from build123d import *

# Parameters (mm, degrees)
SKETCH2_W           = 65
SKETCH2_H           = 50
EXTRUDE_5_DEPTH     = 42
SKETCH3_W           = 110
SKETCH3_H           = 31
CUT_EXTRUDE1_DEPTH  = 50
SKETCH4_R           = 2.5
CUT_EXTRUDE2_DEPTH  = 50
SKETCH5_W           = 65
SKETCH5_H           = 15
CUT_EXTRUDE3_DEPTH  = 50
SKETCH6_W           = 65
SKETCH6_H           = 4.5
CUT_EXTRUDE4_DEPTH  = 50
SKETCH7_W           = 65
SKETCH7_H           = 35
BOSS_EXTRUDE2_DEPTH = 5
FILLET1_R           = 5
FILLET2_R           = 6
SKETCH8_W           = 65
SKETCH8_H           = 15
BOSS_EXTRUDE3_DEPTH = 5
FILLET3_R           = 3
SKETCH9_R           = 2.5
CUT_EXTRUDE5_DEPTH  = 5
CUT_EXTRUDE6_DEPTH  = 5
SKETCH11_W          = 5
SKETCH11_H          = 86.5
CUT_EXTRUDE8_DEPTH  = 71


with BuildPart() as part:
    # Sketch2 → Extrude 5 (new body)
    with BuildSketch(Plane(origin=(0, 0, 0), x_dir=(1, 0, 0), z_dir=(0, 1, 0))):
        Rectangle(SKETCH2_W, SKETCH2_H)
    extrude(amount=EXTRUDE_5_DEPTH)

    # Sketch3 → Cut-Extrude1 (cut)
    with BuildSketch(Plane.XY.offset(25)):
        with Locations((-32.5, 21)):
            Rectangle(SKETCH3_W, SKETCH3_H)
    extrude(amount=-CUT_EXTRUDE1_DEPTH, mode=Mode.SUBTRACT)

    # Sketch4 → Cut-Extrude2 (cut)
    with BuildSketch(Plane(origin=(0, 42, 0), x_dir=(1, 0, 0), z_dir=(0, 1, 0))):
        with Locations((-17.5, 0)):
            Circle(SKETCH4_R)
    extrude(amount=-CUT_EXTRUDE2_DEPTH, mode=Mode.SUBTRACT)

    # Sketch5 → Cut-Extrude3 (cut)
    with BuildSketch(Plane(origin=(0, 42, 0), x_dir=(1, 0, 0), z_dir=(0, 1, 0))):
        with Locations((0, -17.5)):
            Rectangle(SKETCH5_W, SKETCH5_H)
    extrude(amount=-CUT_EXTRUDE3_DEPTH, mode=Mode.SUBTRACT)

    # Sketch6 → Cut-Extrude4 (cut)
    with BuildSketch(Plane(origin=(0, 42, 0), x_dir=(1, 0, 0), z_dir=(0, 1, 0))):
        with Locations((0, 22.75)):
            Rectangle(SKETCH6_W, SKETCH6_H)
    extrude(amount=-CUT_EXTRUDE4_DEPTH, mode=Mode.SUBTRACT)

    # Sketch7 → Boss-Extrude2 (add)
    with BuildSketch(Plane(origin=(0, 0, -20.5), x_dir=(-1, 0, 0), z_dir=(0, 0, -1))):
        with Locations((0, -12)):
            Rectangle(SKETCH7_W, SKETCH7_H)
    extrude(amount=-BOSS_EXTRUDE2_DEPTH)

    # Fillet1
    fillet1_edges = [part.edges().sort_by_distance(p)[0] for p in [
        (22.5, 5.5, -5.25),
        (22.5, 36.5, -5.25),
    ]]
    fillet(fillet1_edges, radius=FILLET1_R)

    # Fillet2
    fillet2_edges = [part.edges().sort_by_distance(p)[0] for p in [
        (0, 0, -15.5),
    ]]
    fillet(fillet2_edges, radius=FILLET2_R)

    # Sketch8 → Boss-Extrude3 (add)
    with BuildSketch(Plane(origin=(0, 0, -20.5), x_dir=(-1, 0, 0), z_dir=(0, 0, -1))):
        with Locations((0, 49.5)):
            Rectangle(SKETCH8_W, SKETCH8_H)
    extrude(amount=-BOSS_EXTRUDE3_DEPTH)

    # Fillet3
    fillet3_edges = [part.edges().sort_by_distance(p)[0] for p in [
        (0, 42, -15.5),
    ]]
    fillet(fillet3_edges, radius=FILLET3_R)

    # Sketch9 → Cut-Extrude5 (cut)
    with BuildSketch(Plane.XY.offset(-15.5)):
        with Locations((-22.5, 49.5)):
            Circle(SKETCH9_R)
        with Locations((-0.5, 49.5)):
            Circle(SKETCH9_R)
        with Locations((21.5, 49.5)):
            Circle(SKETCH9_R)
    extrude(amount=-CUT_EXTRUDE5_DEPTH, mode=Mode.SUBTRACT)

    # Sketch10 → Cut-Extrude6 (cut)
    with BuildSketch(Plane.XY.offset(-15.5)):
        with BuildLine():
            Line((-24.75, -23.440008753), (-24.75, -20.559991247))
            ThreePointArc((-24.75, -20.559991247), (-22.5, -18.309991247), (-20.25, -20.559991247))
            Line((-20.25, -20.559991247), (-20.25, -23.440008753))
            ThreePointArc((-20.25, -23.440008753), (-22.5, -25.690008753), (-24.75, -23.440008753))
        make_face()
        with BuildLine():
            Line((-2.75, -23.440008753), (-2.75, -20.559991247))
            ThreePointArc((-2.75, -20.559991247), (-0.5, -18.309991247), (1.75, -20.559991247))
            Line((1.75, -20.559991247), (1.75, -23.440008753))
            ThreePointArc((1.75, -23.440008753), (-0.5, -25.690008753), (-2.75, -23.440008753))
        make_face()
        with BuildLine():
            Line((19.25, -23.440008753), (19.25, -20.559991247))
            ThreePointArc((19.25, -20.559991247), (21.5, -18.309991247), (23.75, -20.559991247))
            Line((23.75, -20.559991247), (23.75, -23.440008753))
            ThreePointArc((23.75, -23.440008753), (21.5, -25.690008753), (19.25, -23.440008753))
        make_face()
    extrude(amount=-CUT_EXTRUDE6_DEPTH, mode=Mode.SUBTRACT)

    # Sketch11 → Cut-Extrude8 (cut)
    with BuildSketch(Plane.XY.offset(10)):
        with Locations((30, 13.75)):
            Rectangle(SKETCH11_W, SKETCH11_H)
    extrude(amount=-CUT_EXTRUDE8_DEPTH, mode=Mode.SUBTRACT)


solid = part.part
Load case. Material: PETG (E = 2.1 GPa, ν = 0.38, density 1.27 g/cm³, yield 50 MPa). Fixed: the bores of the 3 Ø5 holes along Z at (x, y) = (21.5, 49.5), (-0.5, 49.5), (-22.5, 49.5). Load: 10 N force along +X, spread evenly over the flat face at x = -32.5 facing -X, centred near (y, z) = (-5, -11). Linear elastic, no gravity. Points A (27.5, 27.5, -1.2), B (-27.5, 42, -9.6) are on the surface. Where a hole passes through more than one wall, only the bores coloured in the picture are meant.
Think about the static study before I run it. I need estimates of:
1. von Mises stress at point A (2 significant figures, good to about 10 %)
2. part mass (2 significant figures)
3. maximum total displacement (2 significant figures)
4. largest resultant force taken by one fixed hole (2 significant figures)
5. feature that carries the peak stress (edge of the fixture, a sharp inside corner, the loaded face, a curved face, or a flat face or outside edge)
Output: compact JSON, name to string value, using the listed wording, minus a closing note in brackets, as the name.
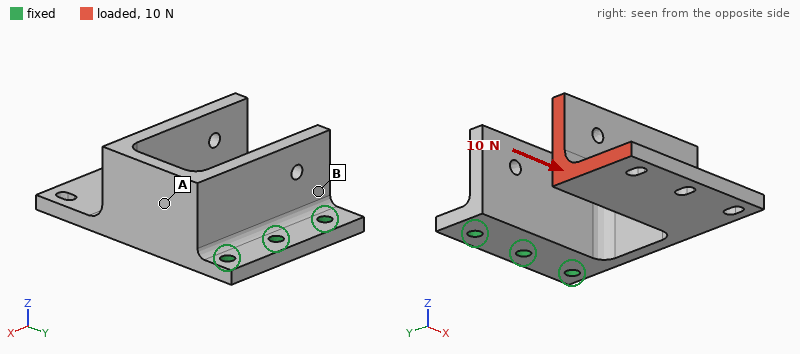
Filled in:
{"von Mises stress at point A": "2.1 MPa", "part mass": "48 g", "maximum total displacement": "1.1 mm", "largest resultant force taken by one fixed hole": "21 N", "feature that carries the peak stress": "a curved face"}
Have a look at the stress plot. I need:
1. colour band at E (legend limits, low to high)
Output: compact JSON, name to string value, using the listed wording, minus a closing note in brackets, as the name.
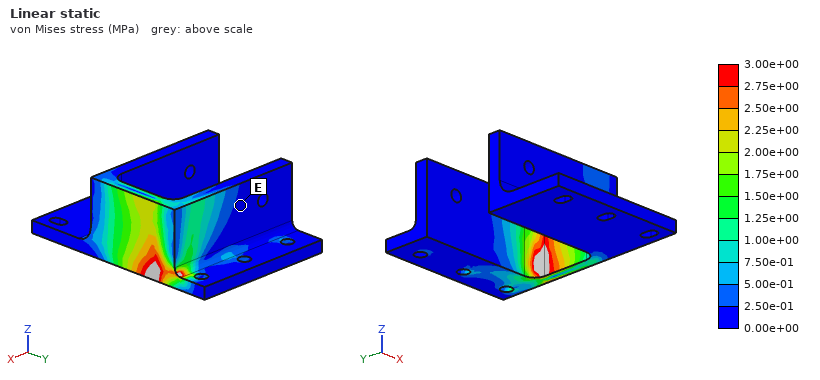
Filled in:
{"colour band at E": "0.00e+00 to 2.50e-01 MPa"}
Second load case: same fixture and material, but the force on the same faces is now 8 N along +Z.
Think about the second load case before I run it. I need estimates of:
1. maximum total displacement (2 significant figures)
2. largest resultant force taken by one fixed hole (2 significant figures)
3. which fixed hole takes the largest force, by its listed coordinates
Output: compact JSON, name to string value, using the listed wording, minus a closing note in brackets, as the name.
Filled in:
{"maximum total displacement": "1.1 mm", "largest resultant force taken by one fixed hole": "11 N", "which fixed hole takes the largest force, by its listed coordinates": "(-0.5, 49.5)"}
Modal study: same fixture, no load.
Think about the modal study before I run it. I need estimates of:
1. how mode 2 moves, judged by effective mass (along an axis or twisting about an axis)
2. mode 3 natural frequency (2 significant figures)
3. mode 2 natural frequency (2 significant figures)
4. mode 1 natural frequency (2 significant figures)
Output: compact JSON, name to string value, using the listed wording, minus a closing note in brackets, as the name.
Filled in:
{"how mode 2 moves, judged by effective mass": "along Z", "mode 3 natural frequency": "340 Hz", "mode 2 natural frequency": "130 Hz", "mode 1 natural frequency": "100 Hz"}
